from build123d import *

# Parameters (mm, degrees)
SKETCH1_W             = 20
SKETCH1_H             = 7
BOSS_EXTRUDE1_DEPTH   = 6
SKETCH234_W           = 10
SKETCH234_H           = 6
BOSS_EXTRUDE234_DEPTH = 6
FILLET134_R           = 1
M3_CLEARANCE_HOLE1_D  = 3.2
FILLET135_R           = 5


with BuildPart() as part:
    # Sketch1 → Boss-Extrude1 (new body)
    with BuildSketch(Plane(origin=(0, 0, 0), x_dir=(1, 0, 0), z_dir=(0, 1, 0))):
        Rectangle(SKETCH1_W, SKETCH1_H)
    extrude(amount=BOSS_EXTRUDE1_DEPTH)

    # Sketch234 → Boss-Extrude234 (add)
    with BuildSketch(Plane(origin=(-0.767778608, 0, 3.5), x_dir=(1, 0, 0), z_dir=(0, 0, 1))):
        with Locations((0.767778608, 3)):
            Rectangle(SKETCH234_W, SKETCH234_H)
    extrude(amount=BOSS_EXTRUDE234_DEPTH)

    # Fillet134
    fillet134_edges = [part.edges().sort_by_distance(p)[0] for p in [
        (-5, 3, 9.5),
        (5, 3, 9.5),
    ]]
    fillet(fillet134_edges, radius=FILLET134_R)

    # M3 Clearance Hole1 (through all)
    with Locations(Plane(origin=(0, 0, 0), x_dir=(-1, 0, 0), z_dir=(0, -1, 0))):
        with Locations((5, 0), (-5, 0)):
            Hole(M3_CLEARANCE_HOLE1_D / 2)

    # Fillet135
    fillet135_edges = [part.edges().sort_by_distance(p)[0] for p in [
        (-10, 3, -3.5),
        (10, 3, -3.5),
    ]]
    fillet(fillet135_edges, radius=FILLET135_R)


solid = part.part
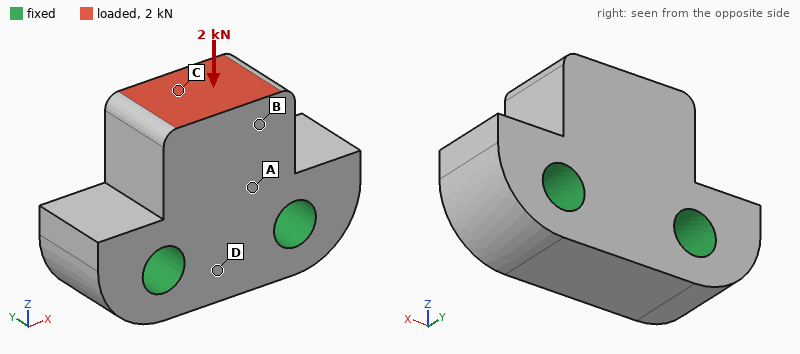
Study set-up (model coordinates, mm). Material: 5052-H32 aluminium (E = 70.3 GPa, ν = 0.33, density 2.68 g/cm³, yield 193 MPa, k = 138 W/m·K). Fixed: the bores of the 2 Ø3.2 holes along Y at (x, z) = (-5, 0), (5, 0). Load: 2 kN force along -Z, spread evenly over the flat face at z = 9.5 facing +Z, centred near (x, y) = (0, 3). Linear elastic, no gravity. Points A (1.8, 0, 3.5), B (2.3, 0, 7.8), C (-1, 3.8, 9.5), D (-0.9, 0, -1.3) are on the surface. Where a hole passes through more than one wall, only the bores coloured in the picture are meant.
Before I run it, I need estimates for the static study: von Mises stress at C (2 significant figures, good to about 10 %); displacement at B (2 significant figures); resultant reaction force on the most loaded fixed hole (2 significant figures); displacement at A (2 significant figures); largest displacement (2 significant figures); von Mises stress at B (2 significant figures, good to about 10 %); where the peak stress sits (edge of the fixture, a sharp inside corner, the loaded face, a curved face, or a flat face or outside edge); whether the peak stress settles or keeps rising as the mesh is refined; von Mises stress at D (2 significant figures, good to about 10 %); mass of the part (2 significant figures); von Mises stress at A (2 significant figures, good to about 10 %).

36 MPa
3.8 µm
1.1 kN
2.0 µm
5.1 µm
42 MPa
edge of the fixture
keeps rising
10.0 MPa
2.8 g
27 MPa
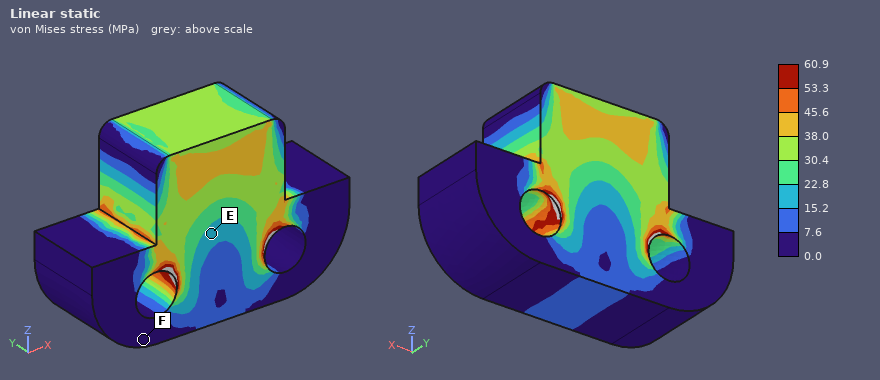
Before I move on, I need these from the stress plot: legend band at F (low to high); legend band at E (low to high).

0.0 to 7.6 MPa
15.2 to 22.8 MPa
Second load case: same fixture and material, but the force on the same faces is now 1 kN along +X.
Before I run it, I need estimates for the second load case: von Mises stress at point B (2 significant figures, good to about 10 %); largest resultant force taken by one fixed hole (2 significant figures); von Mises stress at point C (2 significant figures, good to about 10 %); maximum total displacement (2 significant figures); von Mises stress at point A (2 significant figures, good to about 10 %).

37 MPa
1000 N
37 MPa
9.8 µm
26 MPa
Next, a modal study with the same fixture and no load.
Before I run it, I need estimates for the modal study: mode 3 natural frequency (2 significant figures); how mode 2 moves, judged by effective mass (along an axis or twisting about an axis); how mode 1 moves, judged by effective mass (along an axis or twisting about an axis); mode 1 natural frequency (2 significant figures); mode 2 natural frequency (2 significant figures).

87 kHz
along X
along Y
49 kHz
81 kHz
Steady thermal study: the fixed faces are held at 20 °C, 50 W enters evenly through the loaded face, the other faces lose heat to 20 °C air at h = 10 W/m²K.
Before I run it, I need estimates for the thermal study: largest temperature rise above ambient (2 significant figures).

55 K
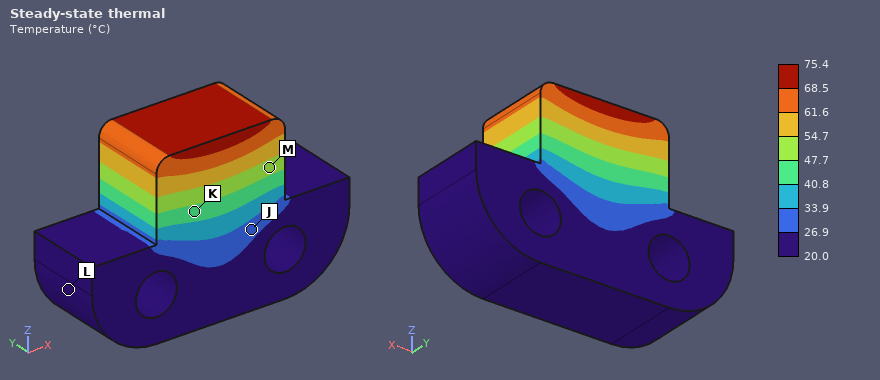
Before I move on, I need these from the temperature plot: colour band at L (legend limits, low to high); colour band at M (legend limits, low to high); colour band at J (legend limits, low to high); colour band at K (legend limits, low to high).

20.0 to 26.9 °C
47.7 to 54.7 °C
26.9 to 33.9 °C
40.8 to 47.7 °C
